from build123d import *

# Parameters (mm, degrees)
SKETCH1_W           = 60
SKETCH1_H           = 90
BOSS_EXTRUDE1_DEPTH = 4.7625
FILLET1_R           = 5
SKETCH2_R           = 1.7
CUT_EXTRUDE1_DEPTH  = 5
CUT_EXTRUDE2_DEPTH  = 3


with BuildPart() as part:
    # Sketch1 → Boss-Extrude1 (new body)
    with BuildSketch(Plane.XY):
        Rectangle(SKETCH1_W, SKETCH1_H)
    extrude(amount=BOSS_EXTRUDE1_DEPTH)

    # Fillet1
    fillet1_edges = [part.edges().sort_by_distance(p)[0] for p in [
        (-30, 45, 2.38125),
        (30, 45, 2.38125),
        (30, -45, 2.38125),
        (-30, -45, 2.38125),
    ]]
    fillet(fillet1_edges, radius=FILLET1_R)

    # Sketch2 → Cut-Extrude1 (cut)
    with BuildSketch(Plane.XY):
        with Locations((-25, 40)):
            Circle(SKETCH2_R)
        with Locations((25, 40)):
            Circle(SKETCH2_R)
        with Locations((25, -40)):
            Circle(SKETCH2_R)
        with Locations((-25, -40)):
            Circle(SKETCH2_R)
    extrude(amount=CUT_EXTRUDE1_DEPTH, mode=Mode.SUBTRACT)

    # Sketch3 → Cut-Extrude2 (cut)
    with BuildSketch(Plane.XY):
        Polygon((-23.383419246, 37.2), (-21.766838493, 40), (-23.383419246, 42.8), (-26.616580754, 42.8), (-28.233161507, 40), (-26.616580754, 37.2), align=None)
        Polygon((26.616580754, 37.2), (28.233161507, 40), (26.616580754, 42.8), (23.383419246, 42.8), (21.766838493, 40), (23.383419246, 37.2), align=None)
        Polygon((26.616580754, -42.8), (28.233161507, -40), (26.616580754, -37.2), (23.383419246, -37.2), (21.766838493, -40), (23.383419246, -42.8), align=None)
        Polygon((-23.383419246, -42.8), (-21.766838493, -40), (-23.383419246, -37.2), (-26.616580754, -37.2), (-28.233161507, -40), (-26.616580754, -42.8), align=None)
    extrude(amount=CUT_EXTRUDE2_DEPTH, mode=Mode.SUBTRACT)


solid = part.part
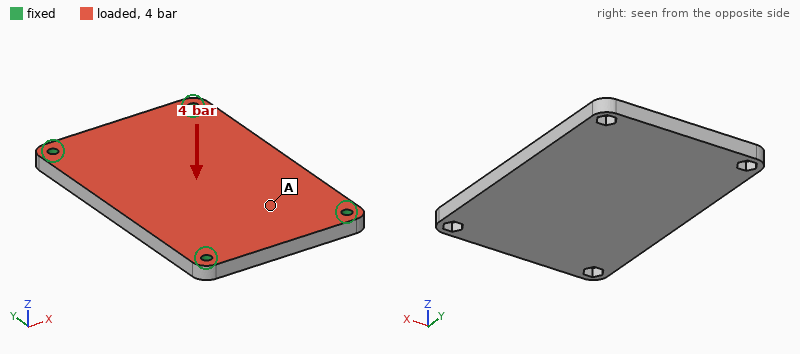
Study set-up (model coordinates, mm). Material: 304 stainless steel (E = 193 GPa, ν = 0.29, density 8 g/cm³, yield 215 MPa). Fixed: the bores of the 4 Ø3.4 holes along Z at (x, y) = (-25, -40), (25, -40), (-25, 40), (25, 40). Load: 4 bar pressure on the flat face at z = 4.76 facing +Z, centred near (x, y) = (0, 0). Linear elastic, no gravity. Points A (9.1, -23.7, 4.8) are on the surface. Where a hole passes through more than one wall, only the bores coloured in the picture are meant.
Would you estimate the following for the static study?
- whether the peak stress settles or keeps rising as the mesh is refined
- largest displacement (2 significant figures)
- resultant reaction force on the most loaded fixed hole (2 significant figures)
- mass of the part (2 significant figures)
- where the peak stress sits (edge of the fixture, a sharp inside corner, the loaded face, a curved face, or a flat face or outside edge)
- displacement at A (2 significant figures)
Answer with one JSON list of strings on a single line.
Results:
["keeps rising", "59 µm", "1.1 kN", "200 g", "edge of the fixture", "37 µm"]
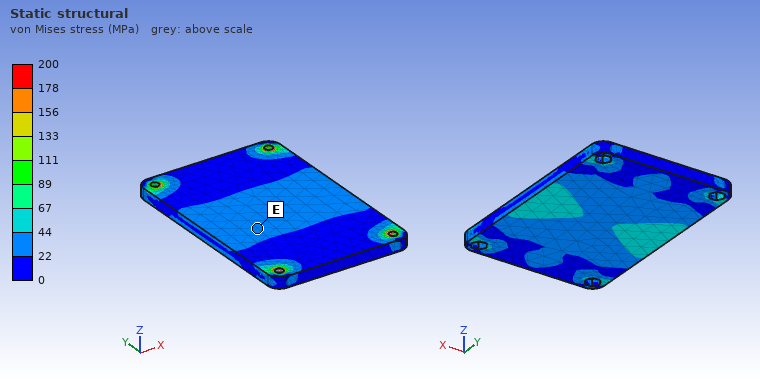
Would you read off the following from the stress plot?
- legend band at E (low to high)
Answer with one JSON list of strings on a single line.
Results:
["22 to 44 MPa"]
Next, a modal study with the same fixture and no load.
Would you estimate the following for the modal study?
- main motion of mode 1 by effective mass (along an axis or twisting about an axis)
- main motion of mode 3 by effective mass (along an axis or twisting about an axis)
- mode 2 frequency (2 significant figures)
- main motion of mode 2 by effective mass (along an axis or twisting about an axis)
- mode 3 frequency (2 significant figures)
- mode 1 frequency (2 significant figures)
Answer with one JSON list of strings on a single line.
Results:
["along Z", "twisting about X", "4200 Hz", "twisting about Y", "6100 Hz", "2400 Hz"]
